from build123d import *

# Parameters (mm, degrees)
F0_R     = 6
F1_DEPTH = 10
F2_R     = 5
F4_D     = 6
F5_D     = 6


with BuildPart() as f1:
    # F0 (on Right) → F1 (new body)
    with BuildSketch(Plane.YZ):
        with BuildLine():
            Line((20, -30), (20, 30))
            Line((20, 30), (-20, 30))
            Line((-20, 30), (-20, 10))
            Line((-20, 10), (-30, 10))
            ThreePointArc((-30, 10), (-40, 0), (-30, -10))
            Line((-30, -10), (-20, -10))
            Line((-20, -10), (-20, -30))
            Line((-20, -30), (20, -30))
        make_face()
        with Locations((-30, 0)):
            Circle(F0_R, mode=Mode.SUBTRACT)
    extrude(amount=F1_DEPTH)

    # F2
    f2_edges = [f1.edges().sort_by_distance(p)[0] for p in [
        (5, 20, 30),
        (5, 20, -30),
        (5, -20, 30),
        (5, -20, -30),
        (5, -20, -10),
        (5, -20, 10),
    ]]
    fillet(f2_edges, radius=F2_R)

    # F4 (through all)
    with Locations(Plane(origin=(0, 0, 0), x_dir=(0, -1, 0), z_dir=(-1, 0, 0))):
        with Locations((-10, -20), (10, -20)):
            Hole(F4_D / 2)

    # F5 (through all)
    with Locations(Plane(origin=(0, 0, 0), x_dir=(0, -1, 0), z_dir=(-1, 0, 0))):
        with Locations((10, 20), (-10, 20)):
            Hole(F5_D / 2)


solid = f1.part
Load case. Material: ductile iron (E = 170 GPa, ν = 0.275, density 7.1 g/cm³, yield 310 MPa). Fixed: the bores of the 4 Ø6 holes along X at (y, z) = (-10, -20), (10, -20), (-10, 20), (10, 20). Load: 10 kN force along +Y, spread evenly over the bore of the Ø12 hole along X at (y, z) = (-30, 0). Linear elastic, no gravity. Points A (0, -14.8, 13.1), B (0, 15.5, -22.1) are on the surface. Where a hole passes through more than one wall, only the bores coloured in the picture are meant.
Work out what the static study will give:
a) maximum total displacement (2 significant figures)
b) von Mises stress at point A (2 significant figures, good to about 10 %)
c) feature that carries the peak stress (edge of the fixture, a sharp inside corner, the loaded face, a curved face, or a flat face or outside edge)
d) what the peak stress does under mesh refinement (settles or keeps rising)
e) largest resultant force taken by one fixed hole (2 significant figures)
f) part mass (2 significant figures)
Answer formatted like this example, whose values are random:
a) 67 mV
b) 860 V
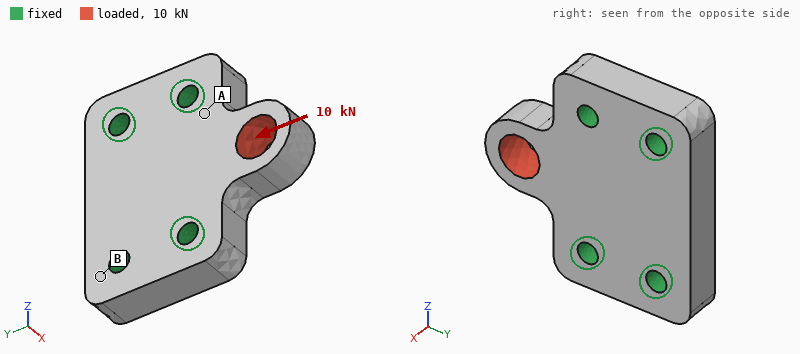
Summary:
a) 16 µm
b) 44 MPa
c) a sharp inside corner
d) keeps rising
e) 3.4 kN
f) 180 g
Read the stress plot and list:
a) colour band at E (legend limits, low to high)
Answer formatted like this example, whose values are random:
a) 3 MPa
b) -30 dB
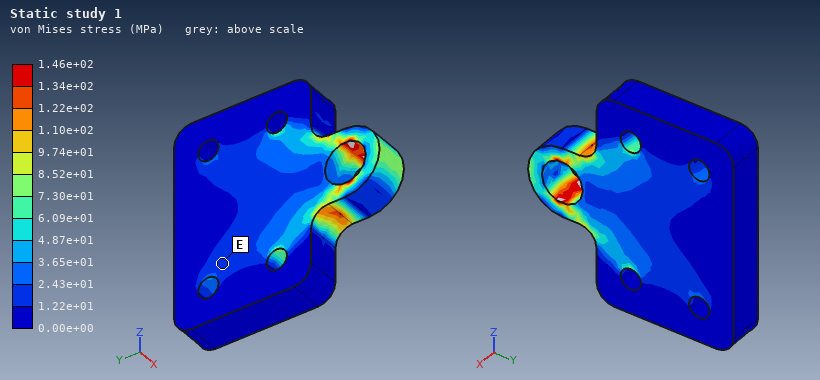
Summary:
a) 1.22e+01 to 2.43e+01 MPa
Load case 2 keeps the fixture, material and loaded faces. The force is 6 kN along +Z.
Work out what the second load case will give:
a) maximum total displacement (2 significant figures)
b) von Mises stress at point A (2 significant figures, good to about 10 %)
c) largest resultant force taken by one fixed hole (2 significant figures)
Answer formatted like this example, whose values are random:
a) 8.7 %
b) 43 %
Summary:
a) 39 µm
b) 46 MPa
c) 3.9 kN
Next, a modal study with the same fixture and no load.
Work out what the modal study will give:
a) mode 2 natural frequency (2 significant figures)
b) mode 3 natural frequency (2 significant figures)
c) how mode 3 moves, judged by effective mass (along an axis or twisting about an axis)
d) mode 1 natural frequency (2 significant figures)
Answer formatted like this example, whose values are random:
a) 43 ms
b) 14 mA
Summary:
a) 18 kHz
b) 24 kHz
c) along X
d) 10 kHz
